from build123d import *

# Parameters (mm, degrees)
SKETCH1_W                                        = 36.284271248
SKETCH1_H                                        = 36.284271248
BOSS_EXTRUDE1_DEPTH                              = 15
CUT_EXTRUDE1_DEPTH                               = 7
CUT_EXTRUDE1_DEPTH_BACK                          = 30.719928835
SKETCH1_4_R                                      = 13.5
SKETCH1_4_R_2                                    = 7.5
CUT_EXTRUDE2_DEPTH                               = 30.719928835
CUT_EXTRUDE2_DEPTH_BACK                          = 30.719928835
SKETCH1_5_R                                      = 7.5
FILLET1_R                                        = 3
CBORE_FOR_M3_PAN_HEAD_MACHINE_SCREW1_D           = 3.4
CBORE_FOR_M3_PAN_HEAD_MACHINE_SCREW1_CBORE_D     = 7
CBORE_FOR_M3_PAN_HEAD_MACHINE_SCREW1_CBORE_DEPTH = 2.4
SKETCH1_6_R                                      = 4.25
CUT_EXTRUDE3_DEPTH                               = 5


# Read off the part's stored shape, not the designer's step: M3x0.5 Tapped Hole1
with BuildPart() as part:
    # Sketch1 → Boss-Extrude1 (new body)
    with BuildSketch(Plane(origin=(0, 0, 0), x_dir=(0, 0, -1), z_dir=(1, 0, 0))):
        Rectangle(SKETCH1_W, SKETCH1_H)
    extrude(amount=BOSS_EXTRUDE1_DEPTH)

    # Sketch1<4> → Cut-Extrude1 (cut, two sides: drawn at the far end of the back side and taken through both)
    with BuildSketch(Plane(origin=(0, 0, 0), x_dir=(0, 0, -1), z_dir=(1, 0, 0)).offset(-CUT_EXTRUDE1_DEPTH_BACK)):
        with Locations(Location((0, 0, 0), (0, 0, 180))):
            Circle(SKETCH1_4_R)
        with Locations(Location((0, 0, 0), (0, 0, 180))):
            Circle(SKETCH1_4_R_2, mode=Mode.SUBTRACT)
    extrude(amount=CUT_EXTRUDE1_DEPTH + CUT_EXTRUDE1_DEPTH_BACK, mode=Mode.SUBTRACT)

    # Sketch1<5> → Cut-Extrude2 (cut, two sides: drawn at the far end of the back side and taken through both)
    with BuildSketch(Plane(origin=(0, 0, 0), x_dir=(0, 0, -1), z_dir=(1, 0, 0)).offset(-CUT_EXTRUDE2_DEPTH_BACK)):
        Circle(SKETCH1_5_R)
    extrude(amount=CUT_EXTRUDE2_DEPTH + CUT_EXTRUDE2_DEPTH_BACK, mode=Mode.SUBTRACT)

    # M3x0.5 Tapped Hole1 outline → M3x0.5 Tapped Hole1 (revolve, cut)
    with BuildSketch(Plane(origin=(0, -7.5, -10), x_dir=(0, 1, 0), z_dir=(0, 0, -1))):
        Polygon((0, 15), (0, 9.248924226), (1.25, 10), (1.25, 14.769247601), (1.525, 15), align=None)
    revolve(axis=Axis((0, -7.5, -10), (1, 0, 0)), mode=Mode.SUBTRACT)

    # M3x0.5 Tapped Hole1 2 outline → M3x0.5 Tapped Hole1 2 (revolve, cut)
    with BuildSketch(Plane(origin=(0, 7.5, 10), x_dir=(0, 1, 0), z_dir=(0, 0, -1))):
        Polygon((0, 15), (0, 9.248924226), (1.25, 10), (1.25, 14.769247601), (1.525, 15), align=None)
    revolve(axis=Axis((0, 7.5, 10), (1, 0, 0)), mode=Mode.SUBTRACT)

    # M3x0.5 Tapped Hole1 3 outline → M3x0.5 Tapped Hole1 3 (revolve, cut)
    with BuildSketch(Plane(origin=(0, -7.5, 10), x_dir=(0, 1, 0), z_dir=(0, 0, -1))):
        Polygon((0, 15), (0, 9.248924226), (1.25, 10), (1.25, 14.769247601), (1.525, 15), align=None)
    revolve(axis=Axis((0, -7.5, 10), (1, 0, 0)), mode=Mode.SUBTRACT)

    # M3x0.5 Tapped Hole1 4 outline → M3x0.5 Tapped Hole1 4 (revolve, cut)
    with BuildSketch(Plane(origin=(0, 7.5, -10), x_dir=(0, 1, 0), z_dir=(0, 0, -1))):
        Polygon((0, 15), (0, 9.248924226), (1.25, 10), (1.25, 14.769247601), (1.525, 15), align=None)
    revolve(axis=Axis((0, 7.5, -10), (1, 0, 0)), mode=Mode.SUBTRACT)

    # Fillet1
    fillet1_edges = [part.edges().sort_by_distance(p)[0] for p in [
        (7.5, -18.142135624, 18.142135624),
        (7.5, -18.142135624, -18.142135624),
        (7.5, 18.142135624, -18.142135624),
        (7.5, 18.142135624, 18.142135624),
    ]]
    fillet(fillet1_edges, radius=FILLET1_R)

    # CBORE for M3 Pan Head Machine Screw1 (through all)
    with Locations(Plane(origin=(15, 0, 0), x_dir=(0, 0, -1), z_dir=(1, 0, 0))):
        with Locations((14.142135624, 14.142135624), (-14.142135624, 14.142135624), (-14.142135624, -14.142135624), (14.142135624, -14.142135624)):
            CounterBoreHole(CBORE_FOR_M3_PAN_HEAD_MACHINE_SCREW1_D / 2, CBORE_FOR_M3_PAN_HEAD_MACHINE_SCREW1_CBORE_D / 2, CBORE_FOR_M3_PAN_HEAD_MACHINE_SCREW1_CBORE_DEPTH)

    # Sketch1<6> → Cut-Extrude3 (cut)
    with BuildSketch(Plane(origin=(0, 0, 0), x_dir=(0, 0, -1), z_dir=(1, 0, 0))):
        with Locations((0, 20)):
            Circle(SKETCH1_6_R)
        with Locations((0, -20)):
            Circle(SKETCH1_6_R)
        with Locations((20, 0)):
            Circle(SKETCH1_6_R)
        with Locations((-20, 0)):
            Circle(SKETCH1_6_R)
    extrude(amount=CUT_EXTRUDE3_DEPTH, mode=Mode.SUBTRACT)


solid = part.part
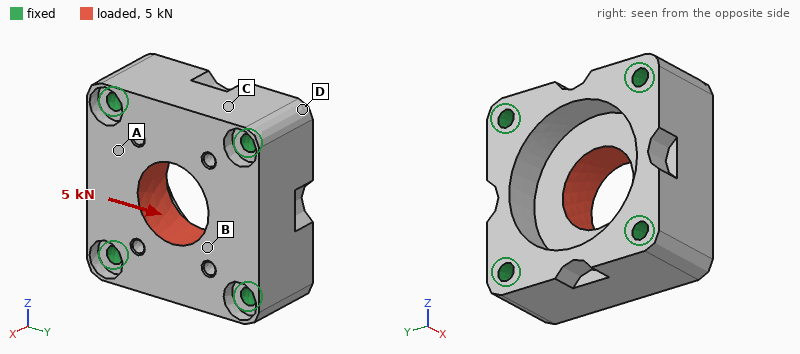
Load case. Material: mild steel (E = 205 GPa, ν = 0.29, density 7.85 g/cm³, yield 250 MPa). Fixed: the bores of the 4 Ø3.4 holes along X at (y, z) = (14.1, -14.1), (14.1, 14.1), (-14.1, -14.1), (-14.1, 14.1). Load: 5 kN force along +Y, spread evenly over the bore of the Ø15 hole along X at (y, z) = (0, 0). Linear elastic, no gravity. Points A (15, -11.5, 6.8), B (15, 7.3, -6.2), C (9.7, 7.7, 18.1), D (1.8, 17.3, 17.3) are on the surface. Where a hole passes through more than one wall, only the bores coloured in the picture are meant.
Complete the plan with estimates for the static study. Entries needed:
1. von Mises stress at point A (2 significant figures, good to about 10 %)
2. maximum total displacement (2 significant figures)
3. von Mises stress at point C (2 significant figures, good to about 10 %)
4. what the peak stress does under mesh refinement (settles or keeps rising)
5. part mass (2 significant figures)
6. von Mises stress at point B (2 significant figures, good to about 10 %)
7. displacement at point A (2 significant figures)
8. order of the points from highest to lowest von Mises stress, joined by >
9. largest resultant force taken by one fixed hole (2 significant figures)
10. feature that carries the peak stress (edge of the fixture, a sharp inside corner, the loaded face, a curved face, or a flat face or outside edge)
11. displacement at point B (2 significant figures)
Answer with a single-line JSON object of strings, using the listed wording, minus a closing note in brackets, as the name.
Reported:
{"von Mises stress at point A": "14 MPa", "maximum total displacement": "2.0 µm", "von Mises stress at point C": "6.5 MPa", "what the peak stress does under mesh refinement": "keeps rising", "part mass": "100 g", "von Mises stress at point B": "18 MPa", "displacement at point A": "1.2 µm", "order of the points from highest to lowest von Mises stress, joined by >": "B > A > C > D", "largest resultant force taken by one fixed hole": "1.3 kN", "feature that carries the peak stress": "edge of the fixture", "displacement at point B": "1.3 µm"}
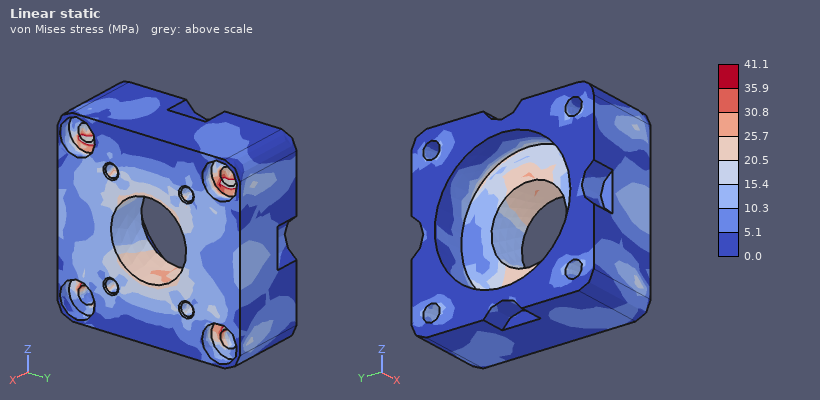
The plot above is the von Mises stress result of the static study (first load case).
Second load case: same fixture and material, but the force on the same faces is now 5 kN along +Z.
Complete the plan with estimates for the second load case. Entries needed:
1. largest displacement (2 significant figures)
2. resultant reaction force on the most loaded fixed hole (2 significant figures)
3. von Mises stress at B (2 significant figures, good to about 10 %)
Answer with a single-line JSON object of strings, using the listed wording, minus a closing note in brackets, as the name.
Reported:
{"largest displacement": "2.0 µm", "resultant reaction force on the most loaded fixed hole": "1.3 kN", "von Mises stress at B": "18 MPa"}
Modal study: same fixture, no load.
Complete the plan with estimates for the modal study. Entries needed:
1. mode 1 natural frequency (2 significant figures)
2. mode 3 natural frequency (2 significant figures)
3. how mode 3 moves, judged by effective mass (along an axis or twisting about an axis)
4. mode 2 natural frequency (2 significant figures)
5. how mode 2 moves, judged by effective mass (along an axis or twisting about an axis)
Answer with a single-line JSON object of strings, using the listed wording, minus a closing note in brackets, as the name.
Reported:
{"mode 1 natural frequency": "35 kHz", "mode 3 natural frequency": "46 kHz", "how mode 3 moves, judged by effective mass": "along Z", "mode 2 natural frequency": "39 kHz", "how mode 2 moves, judged by effective mass": "along X"}
